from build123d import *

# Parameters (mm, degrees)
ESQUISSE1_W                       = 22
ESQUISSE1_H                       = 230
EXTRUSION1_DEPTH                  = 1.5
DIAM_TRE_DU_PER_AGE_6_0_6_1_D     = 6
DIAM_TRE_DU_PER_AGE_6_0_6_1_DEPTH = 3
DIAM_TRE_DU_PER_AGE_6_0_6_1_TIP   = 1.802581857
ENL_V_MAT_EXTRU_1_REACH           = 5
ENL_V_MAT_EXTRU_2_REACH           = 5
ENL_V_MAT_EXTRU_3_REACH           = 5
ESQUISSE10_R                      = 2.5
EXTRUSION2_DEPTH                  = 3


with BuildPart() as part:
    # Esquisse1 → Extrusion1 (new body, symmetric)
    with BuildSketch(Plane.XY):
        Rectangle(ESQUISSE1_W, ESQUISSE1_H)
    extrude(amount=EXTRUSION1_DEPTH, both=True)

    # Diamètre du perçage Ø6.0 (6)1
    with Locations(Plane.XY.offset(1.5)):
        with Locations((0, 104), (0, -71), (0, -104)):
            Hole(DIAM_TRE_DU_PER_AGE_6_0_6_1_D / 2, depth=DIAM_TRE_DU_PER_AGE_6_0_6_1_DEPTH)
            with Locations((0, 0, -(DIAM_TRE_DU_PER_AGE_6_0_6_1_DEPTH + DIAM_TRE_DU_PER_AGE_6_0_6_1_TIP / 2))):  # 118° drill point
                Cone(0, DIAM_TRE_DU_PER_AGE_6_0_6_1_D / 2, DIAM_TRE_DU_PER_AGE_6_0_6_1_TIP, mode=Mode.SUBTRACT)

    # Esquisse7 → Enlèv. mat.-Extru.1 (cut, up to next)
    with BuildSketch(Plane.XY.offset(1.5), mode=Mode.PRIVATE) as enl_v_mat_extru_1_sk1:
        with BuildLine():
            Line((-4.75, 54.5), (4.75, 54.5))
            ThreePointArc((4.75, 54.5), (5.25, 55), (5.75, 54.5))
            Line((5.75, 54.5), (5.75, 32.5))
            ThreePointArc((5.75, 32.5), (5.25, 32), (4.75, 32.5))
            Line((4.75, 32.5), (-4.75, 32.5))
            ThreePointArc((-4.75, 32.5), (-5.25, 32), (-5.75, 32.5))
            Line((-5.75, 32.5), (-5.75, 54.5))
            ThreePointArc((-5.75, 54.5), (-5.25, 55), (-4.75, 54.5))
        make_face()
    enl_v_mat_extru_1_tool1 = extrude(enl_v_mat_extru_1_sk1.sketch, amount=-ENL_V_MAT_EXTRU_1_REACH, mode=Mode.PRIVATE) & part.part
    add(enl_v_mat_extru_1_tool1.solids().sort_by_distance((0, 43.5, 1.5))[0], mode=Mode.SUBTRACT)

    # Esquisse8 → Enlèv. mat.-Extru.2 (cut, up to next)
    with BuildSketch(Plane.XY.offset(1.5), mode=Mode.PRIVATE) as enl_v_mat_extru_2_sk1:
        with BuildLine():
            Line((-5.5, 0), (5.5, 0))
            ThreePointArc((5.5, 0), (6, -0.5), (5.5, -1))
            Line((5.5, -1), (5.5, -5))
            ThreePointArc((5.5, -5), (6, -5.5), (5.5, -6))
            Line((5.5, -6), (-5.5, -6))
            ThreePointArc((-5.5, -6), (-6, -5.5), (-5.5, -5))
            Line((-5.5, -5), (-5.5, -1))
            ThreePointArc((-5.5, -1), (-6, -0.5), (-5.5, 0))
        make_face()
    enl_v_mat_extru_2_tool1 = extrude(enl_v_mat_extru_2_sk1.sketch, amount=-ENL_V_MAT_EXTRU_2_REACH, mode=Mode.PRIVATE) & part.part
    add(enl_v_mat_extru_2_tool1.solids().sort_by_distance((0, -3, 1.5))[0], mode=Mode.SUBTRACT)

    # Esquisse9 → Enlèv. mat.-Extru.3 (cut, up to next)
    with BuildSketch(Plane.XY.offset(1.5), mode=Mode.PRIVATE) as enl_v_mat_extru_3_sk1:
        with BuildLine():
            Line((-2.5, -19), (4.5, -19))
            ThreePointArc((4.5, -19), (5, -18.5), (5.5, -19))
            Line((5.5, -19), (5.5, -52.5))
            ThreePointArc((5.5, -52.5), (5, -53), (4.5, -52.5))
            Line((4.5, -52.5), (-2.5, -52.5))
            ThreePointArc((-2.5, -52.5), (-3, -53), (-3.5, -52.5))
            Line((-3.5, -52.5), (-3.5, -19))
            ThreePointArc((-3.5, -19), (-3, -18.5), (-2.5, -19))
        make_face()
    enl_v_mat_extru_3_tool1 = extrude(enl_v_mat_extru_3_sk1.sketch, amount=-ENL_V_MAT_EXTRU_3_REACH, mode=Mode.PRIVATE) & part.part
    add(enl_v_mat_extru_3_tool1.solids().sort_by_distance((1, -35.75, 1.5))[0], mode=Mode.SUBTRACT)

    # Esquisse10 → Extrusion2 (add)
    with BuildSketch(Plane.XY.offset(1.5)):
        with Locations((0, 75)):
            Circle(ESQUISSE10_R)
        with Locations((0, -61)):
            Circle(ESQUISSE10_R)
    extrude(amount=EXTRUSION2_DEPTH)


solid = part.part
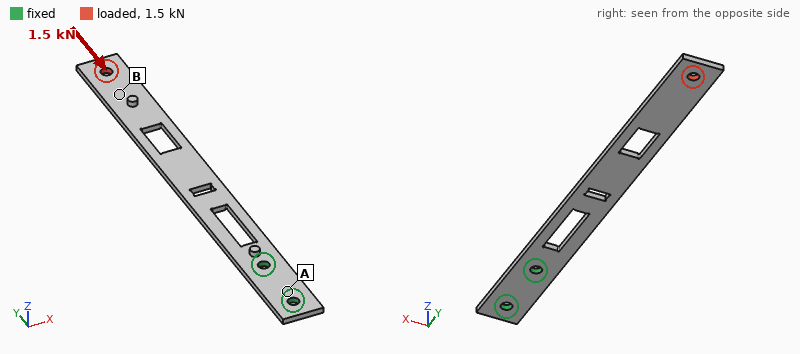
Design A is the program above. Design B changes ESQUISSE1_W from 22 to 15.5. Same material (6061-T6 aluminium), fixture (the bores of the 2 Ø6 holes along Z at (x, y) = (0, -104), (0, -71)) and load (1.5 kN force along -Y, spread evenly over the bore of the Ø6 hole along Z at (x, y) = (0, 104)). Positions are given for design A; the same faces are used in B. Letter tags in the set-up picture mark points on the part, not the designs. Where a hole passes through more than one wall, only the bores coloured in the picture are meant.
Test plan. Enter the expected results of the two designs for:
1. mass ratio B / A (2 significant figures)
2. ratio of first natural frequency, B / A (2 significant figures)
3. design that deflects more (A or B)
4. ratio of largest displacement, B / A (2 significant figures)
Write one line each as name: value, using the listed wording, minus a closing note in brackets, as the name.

mass ratio B / A: 0.66
ratio of first natural frequency, B / A: 0.89
design that deflects more: B
ratio of largest displacement, B / A: 3.3
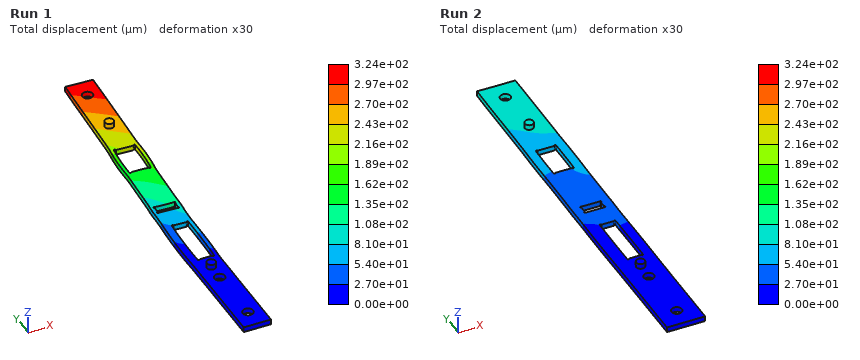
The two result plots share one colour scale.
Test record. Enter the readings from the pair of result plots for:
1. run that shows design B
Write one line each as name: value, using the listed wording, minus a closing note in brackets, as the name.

run that shows design B: Run 1
